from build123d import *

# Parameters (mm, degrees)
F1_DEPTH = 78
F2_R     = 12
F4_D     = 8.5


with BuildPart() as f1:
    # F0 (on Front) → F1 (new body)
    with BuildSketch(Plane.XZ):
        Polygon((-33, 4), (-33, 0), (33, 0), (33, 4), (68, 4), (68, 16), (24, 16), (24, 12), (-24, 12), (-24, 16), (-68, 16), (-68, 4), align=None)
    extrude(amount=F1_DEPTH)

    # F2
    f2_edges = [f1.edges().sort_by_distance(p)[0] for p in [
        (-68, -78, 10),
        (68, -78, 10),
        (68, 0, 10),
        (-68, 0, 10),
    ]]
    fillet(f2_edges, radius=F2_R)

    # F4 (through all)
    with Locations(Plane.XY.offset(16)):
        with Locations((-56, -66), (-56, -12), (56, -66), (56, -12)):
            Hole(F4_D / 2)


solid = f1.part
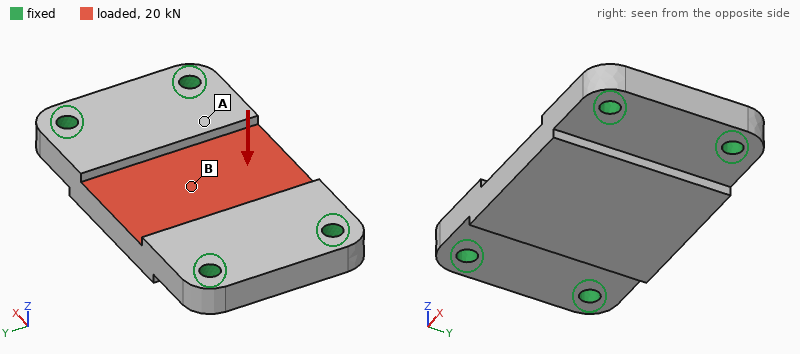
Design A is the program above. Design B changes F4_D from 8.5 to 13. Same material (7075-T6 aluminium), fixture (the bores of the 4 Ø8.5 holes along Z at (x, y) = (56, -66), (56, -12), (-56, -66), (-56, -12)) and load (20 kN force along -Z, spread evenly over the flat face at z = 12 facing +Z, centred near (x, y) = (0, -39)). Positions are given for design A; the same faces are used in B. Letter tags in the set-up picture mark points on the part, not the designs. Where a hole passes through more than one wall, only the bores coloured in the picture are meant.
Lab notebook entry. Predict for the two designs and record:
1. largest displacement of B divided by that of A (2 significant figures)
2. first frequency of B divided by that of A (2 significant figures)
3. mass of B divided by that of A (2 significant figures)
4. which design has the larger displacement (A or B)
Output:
0.82
1.1
0.97
A
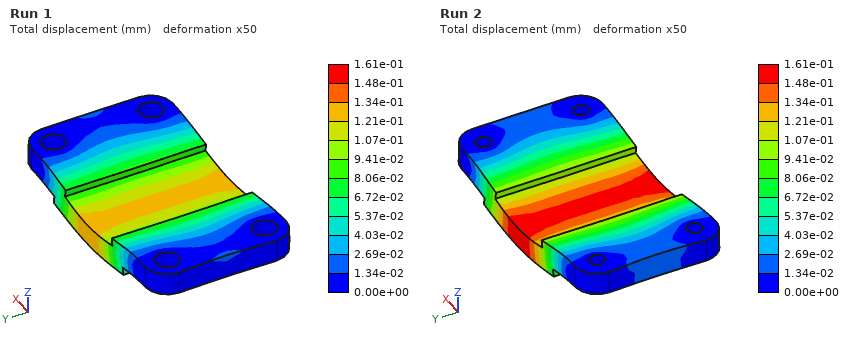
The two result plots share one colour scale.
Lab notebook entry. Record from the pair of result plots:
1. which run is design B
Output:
Run 1
